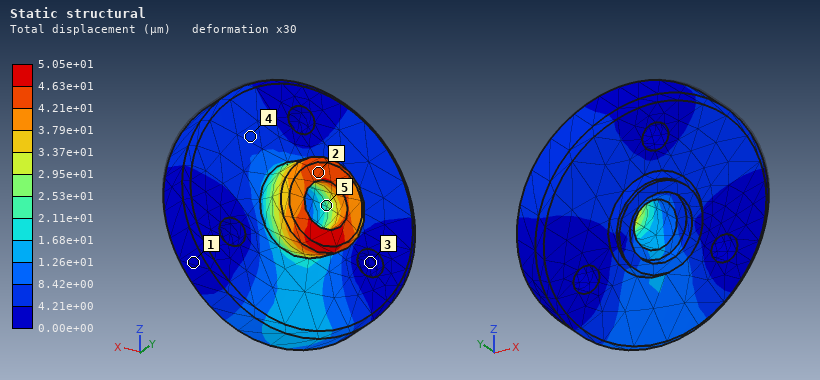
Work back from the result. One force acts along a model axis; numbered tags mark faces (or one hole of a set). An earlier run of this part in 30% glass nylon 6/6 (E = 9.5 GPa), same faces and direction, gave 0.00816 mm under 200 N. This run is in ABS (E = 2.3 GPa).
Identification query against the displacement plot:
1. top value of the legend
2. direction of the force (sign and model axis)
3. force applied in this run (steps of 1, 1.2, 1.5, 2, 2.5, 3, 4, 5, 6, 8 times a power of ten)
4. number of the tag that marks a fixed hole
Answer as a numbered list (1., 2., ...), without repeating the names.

1. 5.05e+01 µm
2. -Z
3. 300 N
4. 3
